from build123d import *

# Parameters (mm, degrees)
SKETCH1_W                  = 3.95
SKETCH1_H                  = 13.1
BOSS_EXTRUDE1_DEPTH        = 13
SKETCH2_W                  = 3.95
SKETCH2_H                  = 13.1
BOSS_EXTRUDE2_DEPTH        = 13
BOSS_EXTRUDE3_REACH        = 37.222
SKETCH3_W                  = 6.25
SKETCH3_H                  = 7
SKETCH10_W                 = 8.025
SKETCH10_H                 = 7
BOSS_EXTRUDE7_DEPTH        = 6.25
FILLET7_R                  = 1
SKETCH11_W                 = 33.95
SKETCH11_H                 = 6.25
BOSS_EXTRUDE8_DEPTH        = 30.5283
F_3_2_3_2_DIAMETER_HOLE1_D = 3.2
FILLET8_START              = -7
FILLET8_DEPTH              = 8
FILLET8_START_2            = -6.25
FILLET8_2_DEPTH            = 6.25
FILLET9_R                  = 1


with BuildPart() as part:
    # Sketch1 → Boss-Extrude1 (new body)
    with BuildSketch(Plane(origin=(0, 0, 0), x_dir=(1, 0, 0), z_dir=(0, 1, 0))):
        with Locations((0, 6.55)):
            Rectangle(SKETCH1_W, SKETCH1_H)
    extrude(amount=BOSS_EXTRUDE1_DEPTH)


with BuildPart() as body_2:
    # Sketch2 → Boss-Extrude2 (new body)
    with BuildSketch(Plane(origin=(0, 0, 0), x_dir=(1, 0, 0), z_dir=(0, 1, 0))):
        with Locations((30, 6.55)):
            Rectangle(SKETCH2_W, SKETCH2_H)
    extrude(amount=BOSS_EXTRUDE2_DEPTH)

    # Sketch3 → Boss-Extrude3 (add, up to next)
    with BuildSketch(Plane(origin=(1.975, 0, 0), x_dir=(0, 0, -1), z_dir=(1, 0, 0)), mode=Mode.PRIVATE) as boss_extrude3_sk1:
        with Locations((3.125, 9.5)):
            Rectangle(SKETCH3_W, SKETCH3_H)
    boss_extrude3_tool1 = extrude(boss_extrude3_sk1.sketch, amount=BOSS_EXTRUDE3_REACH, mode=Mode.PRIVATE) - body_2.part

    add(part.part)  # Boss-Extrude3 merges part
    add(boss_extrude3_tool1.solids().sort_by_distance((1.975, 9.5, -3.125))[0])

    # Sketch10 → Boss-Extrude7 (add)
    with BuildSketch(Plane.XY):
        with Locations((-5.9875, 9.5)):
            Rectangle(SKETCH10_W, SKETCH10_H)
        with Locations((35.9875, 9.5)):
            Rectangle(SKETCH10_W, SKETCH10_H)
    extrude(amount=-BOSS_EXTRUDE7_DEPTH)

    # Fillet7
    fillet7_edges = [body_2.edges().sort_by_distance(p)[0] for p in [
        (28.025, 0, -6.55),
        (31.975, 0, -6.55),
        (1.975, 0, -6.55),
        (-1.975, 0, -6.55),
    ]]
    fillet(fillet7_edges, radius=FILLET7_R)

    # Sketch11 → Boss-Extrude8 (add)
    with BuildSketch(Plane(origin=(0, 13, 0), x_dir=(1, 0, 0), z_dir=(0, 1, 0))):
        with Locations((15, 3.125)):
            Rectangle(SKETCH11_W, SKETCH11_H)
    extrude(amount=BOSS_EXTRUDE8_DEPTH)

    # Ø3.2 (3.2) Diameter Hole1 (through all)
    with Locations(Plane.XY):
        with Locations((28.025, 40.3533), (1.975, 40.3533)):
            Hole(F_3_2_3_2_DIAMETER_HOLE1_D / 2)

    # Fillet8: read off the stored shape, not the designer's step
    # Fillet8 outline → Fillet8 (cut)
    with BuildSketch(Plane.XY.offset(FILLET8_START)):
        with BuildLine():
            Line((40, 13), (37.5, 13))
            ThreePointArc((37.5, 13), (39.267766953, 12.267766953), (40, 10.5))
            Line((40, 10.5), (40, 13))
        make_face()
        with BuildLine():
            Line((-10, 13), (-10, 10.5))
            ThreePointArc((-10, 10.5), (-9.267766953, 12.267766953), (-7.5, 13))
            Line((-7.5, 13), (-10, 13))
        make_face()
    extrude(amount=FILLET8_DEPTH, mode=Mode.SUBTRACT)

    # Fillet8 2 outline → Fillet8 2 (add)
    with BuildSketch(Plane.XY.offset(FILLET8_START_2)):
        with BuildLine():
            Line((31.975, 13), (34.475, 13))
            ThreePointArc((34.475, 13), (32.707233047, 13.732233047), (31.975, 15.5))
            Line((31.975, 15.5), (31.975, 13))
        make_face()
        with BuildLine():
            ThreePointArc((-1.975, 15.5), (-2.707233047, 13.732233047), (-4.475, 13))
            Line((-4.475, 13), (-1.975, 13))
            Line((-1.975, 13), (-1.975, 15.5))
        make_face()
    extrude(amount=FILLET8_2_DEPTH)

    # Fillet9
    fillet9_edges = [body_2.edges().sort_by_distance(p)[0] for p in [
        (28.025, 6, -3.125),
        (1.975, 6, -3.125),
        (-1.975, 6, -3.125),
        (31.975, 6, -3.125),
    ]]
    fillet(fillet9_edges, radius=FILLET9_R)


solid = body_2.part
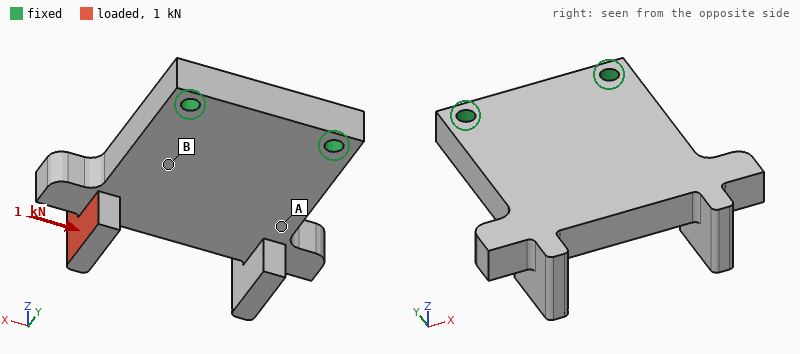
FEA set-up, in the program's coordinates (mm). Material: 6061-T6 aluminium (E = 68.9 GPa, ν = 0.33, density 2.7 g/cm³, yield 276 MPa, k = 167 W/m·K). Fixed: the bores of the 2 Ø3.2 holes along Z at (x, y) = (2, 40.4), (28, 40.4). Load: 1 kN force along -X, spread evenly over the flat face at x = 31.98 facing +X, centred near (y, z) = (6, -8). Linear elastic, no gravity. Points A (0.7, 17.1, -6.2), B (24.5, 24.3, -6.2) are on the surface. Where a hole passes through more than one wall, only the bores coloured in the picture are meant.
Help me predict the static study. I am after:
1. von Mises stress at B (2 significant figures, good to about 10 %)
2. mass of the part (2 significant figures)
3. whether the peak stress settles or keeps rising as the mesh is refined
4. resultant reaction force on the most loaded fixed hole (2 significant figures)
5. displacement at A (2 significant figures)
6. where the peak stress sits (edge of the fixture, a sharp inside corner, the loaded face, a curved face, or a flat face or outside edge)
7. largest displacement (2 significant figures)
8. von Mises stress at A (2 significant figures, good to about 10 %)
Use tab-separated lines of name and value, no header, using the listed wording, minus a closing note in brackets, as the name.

von Mises stress at B	34 MPa
mass of the part	26 g
whether the peak stress settles or keeps rising as the mesh is refined	keeps rising
resultant reaction force on the most loaded fixed hole	1.4 kN
displacement at A	0.020 mm
where the peak stress sits	a sharp inside corner
largest displacement	0.11 mm
von Mises stress at A	12 MPa
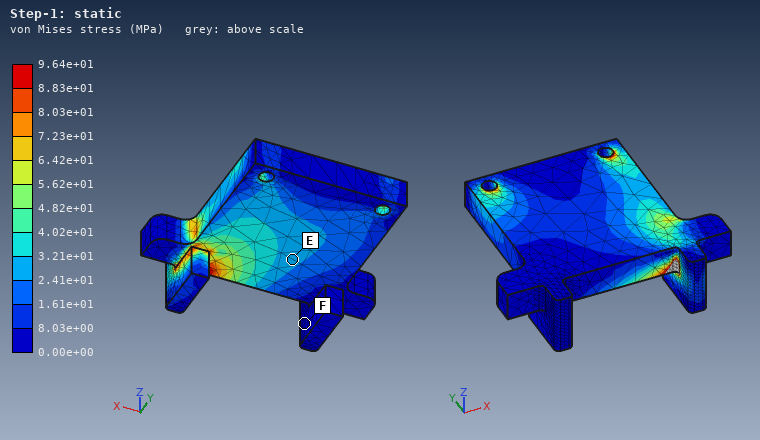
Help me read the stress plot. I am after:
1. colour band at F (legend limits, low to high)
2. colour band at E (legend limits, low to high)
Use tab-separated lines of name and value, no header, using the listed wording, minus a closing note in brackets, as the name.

colour band at F	0.00e+00 to 8.03e+00 MPa
colour band at E	2.41e+01 to 3.21e+01 MPa
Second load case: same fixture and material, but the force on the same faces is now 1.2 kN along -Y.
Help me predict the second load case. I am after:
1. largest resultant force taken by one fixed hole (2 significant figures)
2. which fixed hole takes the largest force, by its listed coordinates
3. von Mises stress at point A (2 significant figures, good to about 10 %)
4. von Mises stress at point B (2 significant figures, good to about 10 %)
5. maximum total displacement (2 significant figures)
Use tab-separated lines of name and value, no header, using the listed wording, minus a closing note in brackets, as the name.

largest resultant force taken by one fixed hole	1.4 kN
which fixed hole takes the largest force, by its listed coordinates	(28, 40.4)
von Mises stress at point A	11 MPa
von Mises stress at point B	48 MPa
maximum total displacement	0.18 mm
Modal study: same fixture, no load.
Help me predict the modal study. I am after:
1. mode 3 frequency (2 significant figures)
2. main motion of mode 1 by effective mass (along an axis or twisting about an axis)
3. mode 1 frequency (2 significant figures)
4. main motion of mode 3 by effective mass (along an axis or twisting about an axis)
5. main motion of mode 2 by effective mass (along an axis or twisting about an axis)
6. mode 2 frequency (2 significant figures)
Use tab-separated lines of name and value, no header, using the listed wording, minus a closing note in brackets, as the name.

mode 3 frequency	11 kHz
main motion of mode 1 by effective mass	along Z
mode 1 frequency	2700 Hz
main motion of mode 3 by effective mass	along X
main motion of mode 2 by effective mass	twisting about Y
mode 2 frequency	5400 Hz
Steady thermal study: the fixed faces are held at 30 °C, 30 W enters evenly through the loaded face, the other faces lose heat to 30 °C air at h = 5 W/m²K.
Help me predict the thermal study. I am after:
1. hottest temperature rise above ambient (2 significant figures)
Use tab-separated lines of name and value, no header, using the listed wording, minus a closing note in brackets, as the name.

hottest temperature rise above ambient	66 K
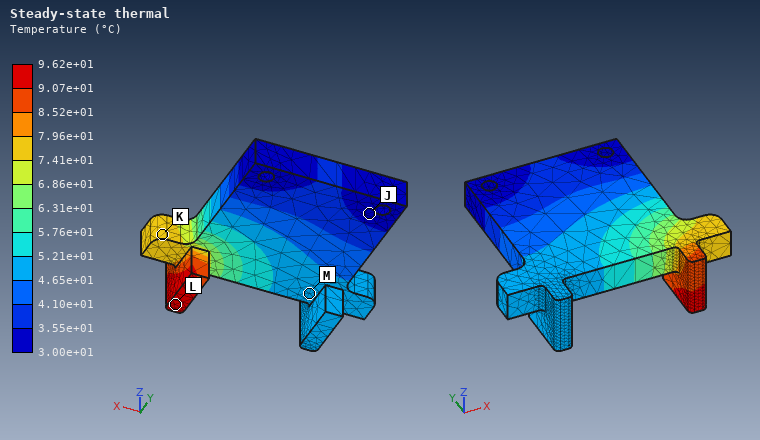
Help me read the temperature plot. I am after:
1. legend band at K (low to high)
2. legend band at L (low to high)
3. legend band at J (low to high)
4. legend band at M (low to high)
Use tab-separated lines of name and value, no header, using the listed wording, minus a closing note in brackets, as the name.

legend band at K	7.41e+01 to 7.96e+01 °C
legend band at L	9.07e+01 to 9.62e+01 °C
legend band at J	3.00e+01 to 3.55e+01 °C
legend band at M	4.65e+01 to 5.21e+01 °C
